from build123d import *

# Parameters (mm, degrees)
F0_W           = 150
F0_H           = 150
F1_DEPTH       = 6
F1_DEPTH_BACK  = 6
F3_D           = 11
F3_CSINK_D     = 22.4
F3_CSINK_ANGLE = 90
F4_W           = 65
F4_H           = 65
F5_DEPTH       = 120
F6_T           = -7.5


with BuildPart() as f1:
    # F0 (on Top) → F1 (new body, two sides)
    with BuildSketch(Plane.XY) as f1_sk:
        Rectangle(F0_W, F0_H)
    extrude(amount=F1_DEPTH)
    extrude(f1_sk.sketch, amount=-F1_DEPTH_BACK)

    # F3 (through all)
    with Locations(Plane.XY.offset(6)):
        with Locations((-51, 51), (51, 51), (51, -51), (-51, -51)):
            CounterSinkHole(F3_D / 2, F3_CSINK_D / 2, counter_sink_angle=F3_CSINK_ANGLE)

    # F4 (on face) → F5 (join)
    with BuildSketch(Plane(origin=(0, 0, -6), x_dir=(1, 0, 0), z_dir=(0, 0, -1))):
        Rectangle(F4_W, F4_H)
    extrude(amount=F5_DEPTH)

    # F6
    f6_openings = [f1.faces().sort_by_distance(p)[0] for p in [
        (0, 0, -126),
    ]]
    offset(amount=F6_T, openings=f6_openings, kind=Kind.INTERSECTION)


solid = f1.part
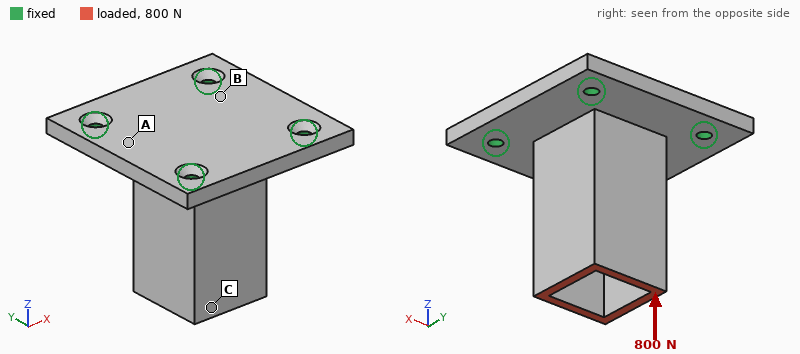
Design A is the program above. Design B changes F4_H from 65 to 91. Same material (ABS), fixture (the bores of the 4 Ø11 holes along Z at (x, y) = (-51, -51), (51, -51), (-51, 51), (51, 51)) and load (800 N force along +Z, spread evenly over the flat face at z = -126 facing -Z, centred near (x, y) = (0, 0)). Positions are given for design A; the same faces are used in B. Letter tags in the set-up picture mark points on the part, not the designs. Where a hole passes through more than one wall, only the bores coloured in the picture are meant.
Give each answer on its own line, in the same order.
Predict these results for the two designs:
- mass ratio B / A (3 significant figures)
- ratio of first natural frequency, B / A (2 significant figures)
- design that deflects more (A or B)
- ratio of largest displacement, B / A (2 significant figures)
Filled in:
1.09
1.1
A
0.70
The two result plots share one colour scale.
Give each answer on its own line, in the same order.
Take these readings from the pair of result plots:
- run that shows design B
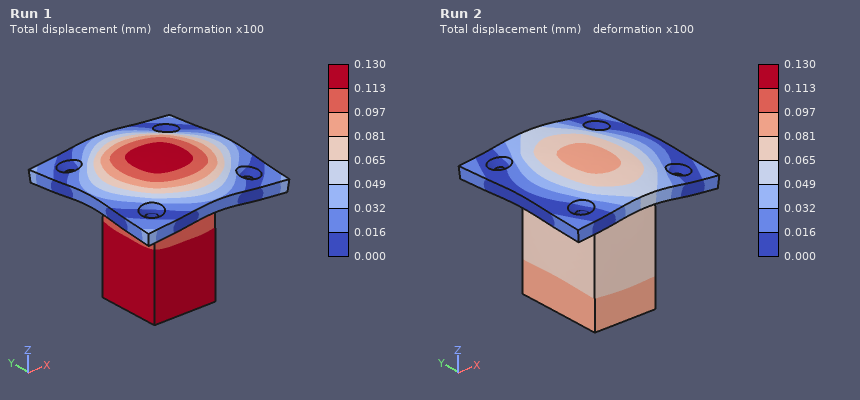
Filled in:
Run 2
